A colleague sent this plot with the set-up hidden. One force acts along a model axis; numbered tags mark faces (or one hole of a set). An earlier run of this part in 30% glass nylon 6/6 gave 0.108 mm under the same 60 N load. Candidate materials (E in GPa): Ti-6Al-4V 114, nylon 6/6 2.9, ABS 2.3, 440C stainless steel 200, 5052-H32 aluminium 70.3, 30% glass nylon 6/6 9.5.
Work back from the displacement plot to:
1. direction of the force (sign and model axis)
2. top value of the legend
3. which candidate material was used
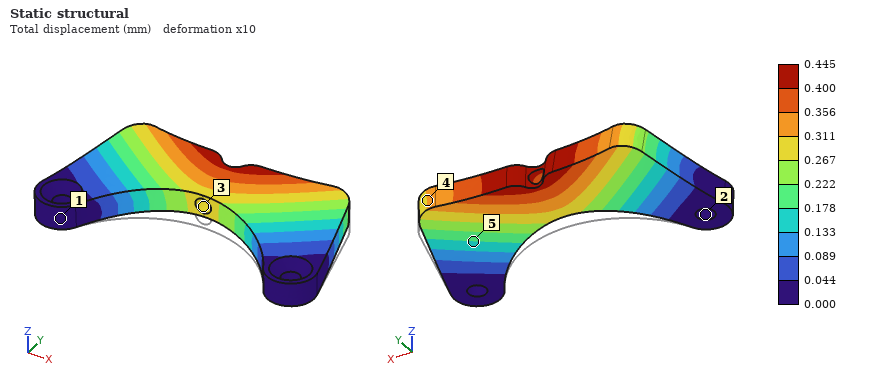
+Z
0.445 mm
ABS
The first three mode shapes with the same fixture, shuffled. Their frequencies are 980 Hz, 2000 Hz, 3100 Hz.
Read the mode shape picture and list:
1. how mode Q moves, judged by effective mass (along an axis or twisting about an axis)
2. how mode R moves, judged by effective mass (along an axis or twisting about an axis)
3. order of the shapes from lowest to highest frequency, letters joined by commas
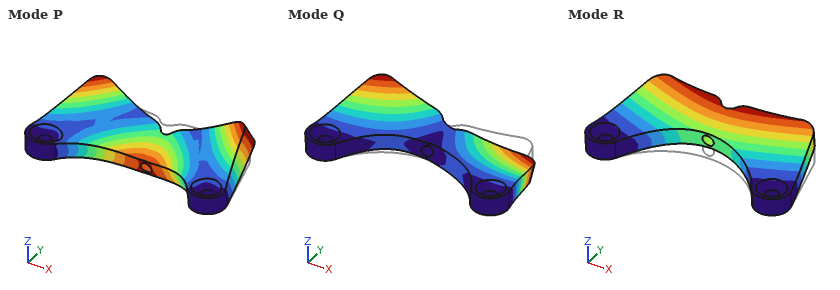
twisting about Y
along Z
R, Q, P
